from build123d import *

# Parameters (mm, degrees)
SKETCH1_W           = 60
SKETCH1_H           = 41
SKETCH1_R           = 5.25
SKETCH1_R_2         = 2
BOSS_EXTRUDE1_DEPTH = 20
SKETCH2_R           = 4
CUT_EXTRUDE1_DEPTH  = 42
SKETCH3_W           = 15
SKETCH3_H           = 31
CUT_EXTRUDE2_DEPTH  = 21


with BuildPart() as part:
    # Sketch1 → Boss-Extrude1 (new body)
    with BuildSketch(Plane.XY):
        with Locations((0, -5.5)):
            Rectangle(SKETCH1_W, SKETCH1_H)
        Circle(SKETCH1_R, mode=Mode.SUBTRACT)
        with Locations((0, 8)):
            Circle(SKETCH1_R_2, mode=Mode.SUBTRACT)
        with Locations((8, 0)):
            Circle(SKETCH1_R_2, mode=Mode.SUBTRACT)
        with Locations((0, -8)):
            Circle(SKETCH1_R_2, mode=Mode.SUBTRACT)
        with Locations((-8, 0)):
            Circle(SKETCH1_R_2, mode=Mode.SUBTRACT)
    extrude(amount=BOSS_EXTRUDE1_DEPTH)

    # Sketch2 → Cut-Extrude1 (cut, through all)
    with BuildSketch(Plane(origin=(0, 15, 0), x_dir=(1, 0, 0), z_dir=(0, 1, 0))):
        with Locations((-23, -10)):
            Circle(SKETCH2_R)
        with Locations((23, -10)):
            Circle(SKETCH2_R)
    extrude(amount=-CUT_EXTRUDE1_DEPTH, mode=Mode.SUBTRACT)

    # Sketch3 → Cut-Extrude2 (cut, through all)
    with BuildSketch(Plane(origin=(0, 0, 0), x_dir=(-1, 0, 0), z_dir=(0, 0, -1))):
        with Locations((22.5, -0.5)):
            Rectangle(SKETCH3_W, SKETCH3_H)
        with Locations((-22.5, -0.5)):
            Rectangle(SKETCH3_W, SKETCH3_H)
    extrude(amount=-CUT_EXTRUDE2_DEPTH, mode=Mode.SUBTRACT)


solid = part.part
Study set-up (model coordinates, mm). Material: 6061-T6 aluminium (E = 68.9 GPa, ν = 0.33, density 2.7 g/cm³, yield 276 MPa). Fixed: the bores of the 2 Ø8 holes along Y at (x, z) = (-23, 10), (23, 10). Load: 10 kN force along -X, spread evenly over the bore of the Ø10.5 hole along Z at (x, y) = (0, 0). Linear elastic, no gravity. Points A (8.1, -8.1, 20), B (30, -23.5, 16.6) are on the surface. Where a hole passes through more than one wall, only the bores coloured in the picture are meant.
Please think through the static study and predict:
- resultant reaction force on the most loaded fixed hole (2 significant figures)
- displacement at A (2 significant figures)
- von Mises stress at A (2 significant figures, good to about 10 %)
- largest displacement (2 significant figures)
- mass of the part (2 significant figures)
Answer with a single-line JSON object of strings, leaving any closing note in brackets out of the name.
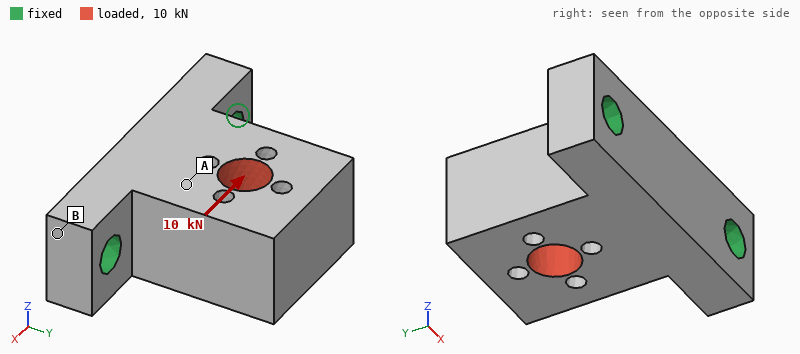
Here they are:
{"resultant reaction force on the most loaded fixed hole": "7.6 kN", "displacement at A": "22 µm", "von Mises stress at A": "43 MPa", "largest displacement": "77 µm", "mass of the part": "73 g"}
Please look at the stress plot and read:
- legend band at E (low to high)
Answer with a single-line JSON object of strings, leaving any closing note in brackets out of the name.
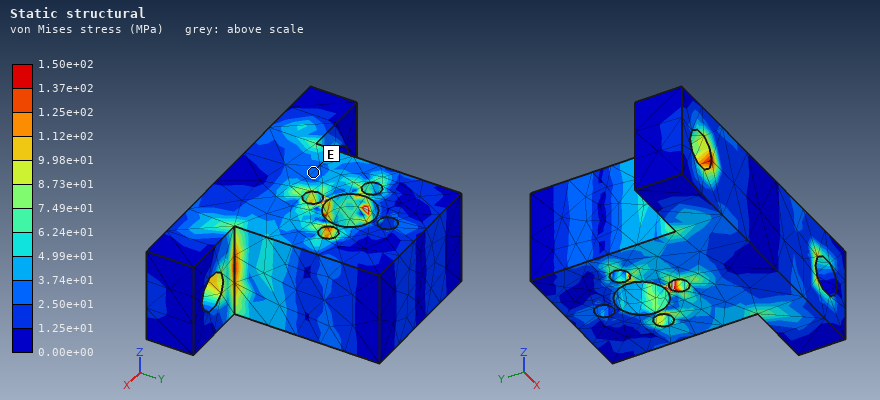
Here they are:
{"legend band at E": "2.50e+01 to 3.74e+01 MPa"}
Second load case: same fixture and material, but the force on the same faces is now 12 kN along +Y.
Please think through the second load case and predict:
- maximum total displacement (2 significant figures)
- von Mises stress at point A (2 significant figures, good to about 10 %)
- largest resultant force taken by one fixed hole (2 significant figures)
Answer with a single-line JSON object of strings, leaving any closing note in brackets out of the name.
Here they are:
{"maximum total displacement": "32 µm", "von Mises stress at point A": "25 MPa", "largest resultant force taken by one fixed hole": "6.4 kN"}
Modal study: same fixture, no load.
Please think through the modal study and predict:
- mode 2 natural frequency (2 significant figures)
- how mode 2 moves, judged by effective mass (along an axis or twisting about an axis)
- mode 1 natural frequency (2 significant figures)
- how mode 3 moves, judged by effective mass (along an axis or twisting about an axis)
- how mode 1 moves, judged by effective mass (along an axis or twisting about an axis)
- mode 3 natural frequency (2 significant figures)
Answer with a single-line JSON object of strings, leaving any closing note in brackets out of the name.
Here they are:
{"mode 2 natural frequency": "10 kHz", "how mode 2 moves, judged by effective mass": "along X", "mode 1 natural frequency": "5100 Hz", "how mode 3 moves, judged by effective mass": "twisting about Y", "how mode 1 moves, judged by effective mass": "along Z", "mode 3 natural frequency": "15 kHz"}
